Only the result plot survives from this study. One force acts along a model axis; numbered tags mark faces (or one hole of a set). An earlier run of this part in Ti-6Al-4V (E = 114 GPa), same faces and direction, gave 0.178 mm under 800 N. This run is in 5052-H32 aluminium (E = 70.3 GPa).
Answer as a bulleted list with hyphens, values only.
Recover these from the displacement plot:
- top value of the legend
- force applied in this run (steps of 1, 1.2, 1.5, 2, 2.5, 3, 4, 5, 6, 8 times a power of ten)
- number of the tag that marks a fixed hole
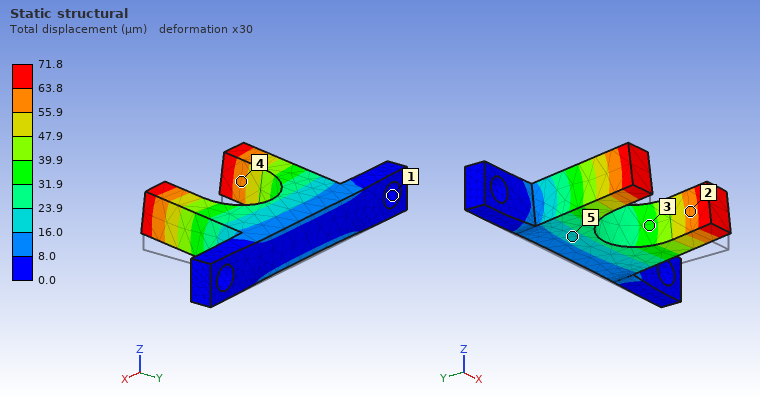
- 71.8 µm
- 200 N
- 1
